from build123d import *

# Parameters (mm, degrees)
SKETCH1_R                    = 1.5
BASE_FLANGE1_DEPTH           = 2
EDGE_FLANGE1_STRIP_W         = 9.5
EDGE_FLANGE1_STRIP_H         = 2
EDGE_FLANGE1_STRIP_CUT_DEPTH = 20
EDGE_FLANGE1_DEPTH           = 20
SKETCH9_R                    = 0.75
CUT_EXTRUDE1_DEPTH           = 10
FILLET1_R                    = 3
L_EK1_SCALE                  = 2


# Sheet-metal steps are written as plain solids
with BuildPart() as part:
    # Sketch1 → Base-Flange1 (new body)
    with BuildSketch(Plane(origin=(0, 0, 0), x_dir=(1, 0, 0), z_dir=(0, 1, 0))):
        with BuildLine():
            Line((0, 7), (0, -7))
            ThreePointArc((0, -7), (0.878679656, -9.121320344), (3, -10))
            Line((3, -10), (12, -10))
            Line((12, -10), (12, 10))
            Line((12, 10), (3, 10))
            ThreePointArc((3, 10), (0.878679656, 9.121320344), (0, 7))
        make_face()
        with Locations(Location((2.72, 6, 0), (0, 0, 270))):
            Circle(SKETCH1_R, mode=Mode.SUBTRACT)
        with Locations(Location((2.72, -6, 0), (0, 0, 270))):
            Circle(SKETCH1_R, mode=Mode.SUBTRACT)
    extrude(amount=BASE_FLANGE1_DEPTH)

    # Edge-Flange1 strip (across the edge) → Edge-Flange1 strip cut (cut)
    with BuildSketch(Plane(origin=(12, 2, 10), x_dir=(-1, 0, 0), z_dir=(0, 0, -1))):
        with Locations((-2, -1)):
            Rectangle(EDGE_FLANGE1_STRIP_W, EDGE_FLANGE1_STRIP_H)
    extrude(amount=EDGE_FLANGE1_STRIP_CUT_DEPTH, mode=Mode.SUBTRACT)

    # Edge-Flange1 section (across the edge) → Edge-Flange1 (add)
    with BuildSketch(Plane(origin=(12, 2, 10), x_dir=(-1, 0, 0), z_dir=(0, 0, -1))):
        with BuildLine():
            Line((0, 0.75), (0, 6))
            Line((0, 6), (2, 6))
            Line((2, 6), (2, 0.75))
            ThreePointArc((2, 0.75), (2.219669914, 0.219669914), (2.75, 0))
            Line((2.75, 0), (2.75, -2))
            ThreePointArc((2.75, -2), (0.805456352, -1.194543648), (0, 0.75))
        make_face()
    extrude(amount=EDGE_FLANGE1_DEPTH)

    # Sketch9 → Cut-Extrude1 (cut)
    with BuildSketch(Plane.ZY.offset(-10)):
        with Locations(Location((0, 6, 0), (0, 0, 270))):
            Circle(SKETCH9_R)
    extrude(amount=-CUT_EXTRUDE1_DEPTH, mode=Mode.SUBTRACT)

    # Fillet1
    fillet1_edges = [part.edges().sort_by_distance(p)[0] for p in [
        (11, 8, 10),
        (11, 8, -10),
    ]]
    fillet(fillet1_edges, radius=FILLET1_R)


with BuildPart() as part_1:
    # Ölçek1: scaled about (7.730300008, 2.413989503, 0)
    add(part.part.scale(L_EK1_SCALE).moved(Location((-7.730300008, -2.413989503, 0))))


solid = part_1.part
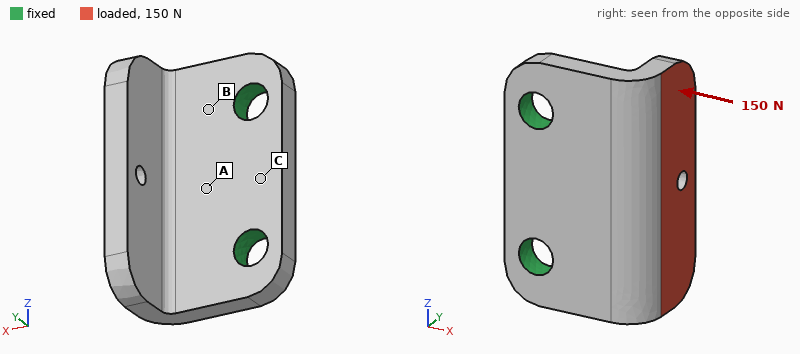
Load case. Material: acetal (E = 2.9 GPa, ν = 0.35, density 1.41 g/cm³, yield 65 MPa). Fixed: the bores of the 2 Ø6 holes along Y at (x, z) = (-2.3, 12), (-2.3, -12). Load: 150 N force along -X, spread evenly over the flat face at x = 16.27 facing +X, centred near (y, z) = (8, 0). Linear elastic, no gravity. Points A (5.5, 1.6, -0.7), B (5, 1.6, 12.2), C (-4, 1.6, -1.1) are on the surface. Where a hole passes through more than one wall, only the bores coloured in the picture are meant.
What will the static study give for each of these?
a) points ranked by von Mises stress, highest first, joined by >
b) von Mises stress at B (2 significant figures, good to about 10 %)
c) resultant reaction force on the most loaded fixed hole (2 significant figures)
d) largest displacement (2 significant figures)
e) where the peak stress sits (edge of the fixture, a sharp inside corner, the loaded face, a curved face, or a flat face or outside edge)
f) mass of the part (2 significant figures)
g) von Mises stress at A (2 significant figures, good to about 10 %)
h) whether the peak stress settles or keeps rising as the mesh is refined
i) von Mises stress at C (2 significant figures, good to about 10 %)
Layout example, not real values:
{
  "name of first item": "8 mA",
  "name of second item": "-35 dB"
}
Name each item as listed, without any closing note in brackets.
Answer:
{
  "points ranked by von Mises stress, highest first, joined by >": "B > A > C",
  "von Mises stress at B": "13 MPa",
  "resultant reaction force on the most loaded fixed hole": "77 N",
  "largest displacement": "0.57 mm",
  "where the peak stress sits": "edge of the fixture",
  "mass of the part": "7.2 g",
  "von Mises stress at A": "10 MPa",
  "whether the peak stress settles or keeps rising as the mesh is refined": "keeps rising",
  "von Mises stress at C": "2.3 MPa"
}
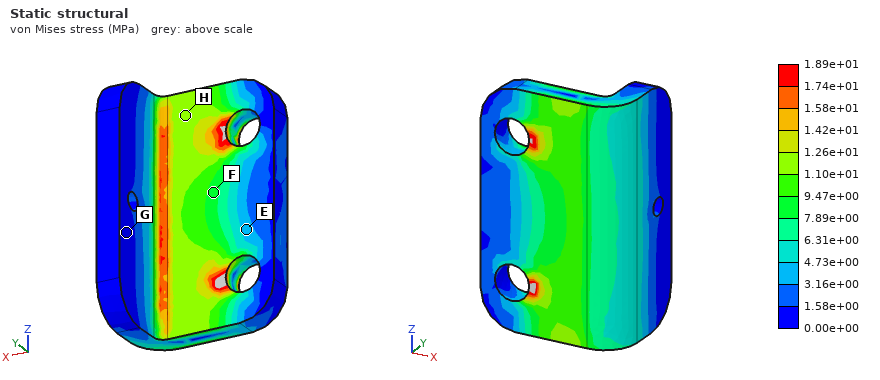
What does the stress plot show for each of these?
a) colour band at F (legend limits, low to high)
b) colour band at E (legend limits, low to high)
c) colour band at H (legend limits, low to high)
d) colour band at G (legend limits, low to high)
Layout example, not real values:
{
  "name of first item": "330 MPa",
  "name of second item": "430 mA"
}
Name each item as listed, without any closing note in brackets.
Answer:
{
  "colour band at F": "7.89e+00 to 9.47e+00 MPa",
  "colour band at E": "3.16e+00 to 4.73e+00 MPa",
  "colour band at H": "1.10e+01 to 1.26e+01 MPa",
  "colour band at G": "0.00e+00 to 1.58e+00 MPa"
}
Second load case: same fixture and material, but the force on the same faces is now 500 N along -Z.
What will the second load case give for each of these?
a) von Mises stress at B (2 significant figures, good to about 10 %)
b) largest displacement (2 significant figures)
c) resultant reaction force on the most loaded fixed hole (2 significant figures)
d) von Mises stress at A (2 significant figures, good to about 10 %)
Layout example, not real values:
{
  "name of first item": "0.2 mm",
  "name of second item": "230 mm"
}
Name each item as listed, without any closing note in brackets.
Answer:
{
  "von Mises stress at B": "17 MPa",
  "largest displacement": "0.52 mm",
  "resultant reaction force on the most loaded fixed hole": "420 N",
  "von Mises stress at A": "17 MPa"
}
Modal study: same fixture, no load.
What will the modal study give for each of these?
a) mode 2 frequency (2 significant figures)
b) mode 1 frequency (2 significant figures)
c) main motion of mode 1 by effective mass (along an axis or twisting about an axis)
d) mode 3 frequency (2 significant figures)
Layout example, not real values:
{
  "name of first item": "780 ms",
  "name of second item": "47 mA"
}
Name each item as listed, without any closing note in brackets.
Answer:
{
  "mode 2 frequency": "2400 Hz",
  "mode 1 frequency": "1500 Hz",
  "main motion of mode 1 by effective mass": "along Y",
  "mode 3 frequency": "4400 Hz"
}
